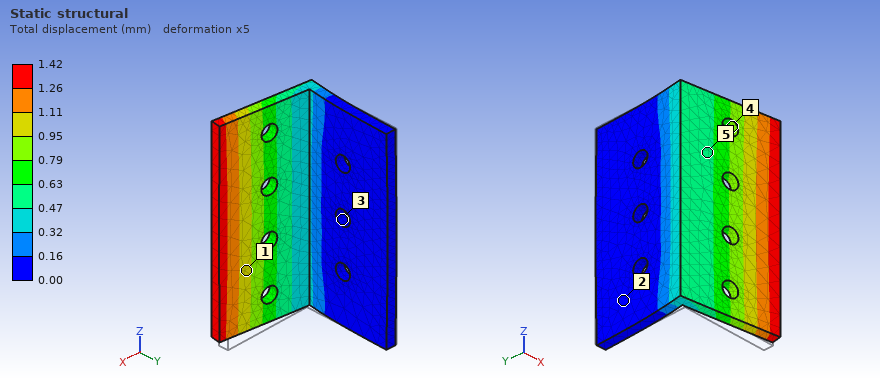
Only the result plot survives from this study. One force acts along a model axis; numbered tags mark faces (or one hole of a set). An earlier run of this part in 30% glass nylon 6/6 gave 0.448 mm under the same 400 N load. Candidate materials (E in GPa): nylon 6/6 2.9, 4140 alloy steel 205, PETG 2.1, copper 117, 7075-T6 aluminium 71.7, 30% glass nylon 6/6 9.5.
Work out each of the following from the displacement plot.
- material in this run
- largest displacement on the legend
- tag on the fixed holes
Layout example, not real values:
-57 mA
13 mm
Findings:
nylon 6/6
1.42 mm
3
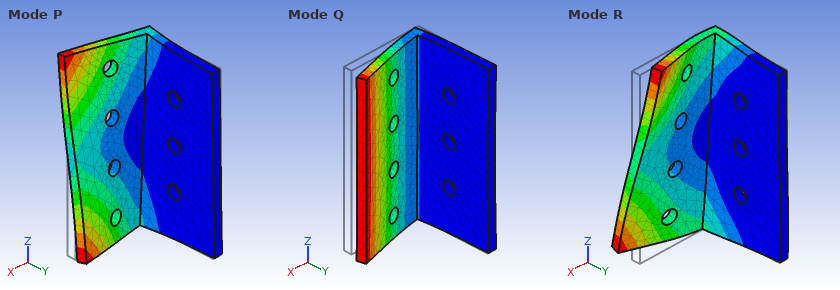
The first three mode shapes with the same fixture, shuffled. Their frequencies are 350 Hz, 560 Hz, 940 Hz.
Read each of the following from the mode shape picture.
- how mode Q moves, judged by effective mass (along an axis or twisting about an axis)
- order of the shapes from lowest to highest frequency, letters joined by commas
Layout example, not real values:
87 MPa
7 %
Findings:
along Y
Q, P, R
